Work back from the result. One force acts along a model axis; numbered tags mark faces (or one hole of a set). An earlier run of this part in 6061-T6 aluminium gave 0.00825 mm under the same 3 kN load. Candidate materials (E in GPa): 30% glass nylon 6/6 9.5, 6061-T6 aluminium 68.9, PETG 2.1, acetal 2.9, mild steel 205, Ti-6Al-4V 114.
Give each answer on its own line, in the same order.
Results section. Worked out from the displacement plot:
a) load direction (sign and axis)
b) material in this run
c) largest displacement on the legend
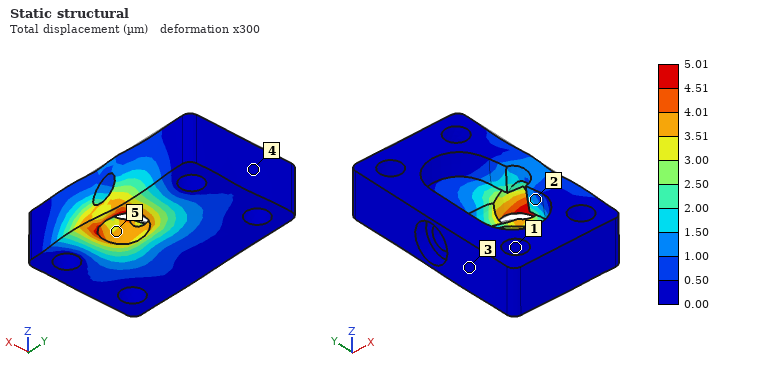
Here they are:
-Y
Ti-6Al-4V
5.01 µm
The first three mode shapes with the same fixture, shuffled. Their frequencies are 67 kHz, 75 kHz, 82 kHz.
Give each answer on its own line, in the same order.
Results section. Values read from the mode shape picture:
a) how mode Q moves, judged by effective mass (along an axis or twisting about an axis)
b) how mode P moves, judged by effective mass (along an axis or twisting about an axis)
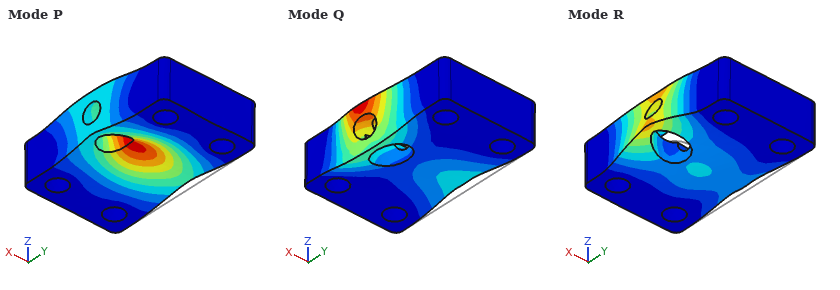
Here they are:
along X
along Z
